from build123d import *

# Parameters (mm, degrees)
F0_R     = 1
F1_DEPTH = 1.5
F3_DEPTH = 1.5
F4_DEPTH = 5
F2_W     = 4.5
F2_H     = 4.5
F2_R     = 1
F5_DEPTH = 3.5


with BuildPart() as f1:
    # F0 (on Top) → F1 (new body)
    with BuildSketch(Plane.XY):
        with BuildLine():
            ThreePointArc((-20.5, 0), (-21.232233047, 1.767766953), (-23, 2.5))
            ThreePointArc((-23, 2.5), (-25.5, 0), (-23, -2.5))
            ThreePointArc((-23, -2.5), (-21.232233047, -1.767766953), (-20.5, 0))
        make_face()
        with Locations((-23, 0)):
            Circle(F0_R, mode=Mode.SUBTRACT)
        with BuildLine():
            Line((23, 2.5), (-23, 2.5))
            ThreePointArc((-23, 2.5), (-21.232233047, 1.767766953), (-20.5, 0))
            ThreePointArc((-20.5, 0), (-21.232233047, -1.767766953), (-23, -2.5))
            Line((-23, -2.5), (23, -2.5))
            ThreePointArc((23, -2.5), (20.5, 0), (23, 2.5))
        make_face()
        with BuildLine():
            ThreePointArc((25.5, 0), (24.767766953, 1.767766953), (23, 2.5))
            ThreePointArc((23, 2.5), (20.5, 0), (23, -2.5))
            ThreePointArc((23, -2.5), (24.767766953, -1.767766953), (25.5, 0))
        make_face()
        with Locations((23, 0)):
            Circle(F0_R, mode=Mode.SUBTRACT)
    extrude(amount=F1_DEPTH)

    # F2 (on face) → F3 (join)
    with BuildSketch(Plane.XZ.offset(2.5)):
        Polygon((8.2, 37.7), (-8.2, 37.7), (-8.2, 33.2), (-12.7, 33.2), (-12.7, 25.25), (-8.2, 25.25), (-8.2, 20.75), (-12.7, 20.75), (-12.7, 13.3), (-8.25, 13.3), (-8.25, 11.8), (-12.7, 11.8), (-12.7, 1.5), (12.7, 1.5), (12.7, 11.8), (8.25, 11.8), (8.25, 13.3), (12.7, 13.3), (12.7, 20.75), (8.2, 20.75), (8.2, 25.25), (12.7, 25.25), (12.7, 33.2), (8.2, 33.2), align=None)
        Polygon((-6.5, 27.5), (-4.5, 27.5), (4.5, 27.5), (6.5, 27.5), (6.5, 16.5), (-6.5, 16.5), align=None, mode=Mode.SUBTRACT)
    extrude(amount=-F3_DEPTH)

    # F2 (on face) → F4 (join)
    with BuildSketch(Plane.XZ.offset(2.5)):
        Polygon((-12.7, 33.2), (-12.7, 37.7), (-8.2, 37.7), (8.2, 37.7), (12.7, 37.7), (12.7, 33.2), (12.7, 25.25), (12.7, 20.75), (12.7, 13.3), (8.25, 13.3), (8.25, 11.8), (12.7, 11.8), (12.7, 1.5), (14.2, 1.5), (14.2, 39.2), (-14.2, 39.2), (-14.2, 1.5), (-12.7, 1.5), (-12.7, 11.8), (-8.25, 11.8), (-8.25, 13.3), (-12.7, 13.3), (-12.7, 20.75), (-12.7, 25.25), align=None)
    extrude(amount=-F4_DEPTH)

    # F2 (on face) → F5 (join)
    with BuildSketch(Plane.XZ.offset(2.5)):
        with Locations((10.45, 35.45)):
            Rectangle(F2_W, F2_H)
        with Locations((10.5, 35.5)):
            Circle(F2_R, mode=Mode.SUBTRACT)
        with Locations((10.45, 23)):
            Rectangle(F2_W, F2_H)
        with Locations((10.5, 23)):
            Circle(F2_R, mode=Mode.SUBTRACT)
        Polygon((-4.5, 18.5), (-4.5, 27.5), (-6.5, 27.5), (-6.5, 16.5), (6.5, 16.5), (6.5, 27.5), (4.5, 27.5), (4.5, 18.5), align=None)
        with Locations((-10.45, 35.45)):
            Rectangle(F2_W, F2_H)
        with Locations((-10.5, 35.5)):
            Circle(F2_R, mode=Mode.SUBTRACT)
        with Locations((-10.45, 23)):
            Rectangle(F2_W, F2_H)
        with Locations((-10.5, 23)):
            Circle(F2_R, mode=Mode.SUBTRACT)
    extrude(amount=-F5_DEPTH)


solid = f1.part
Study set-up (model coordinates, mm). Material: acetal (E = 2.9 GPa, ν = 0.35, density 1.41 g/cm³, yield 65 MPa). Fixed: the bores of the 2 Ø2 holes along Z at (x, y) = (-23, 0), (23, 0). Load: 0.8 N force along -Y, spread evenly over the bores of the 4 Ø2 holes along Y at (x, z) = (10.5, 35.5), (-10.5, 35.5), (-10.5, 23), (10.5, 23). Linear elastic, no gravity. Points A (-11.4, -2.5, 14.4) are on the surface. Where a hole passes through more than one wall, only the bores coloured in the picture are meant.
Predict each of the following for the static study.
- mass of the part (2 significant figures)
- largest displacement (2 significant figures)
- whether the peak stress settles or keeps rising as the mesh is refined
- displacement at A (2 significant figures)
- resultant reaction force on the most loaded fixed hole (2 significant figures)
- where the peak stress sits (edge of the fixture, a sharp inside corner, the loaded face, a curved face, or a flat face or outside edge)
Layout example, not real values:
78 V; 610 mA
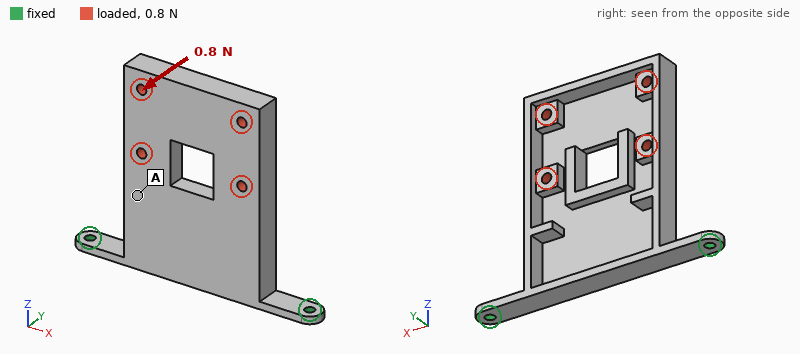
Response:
3.8 g; 0.72 mm; keeps rising; 0.25 mm; 0.51 N; edge of the fixture
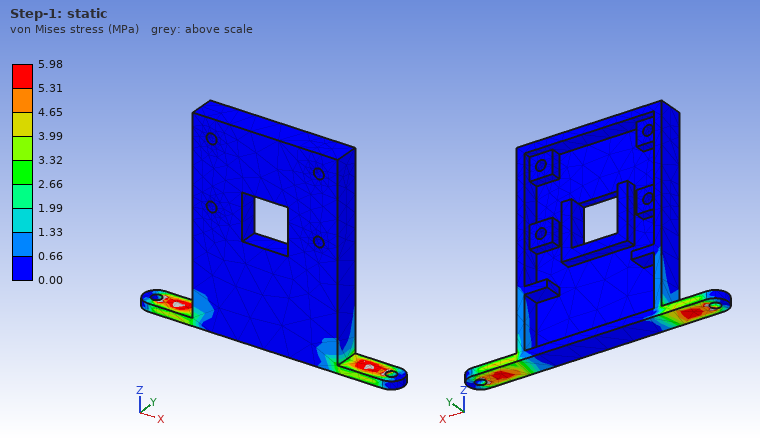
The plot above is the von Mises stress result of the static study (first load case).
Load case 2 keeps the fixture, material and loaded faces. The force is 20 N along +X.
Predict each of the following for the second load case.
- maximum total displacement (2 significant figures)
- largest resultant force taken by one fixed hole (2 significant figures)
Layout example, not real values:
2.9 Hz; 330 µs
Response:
0.72 mm; 19 N
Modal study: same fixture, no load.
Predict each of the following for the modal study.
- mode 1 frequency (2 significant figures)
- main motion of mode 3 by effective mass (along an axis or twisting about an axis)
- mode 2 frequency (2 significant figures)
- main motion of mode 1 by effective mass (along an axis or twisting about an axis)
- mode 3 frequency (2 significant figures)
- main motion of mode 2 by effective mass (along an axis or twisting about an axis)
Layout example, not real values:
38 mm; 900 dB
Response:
130 Hz; along X; 600 Hz; along Y; 730 Hz; along X
